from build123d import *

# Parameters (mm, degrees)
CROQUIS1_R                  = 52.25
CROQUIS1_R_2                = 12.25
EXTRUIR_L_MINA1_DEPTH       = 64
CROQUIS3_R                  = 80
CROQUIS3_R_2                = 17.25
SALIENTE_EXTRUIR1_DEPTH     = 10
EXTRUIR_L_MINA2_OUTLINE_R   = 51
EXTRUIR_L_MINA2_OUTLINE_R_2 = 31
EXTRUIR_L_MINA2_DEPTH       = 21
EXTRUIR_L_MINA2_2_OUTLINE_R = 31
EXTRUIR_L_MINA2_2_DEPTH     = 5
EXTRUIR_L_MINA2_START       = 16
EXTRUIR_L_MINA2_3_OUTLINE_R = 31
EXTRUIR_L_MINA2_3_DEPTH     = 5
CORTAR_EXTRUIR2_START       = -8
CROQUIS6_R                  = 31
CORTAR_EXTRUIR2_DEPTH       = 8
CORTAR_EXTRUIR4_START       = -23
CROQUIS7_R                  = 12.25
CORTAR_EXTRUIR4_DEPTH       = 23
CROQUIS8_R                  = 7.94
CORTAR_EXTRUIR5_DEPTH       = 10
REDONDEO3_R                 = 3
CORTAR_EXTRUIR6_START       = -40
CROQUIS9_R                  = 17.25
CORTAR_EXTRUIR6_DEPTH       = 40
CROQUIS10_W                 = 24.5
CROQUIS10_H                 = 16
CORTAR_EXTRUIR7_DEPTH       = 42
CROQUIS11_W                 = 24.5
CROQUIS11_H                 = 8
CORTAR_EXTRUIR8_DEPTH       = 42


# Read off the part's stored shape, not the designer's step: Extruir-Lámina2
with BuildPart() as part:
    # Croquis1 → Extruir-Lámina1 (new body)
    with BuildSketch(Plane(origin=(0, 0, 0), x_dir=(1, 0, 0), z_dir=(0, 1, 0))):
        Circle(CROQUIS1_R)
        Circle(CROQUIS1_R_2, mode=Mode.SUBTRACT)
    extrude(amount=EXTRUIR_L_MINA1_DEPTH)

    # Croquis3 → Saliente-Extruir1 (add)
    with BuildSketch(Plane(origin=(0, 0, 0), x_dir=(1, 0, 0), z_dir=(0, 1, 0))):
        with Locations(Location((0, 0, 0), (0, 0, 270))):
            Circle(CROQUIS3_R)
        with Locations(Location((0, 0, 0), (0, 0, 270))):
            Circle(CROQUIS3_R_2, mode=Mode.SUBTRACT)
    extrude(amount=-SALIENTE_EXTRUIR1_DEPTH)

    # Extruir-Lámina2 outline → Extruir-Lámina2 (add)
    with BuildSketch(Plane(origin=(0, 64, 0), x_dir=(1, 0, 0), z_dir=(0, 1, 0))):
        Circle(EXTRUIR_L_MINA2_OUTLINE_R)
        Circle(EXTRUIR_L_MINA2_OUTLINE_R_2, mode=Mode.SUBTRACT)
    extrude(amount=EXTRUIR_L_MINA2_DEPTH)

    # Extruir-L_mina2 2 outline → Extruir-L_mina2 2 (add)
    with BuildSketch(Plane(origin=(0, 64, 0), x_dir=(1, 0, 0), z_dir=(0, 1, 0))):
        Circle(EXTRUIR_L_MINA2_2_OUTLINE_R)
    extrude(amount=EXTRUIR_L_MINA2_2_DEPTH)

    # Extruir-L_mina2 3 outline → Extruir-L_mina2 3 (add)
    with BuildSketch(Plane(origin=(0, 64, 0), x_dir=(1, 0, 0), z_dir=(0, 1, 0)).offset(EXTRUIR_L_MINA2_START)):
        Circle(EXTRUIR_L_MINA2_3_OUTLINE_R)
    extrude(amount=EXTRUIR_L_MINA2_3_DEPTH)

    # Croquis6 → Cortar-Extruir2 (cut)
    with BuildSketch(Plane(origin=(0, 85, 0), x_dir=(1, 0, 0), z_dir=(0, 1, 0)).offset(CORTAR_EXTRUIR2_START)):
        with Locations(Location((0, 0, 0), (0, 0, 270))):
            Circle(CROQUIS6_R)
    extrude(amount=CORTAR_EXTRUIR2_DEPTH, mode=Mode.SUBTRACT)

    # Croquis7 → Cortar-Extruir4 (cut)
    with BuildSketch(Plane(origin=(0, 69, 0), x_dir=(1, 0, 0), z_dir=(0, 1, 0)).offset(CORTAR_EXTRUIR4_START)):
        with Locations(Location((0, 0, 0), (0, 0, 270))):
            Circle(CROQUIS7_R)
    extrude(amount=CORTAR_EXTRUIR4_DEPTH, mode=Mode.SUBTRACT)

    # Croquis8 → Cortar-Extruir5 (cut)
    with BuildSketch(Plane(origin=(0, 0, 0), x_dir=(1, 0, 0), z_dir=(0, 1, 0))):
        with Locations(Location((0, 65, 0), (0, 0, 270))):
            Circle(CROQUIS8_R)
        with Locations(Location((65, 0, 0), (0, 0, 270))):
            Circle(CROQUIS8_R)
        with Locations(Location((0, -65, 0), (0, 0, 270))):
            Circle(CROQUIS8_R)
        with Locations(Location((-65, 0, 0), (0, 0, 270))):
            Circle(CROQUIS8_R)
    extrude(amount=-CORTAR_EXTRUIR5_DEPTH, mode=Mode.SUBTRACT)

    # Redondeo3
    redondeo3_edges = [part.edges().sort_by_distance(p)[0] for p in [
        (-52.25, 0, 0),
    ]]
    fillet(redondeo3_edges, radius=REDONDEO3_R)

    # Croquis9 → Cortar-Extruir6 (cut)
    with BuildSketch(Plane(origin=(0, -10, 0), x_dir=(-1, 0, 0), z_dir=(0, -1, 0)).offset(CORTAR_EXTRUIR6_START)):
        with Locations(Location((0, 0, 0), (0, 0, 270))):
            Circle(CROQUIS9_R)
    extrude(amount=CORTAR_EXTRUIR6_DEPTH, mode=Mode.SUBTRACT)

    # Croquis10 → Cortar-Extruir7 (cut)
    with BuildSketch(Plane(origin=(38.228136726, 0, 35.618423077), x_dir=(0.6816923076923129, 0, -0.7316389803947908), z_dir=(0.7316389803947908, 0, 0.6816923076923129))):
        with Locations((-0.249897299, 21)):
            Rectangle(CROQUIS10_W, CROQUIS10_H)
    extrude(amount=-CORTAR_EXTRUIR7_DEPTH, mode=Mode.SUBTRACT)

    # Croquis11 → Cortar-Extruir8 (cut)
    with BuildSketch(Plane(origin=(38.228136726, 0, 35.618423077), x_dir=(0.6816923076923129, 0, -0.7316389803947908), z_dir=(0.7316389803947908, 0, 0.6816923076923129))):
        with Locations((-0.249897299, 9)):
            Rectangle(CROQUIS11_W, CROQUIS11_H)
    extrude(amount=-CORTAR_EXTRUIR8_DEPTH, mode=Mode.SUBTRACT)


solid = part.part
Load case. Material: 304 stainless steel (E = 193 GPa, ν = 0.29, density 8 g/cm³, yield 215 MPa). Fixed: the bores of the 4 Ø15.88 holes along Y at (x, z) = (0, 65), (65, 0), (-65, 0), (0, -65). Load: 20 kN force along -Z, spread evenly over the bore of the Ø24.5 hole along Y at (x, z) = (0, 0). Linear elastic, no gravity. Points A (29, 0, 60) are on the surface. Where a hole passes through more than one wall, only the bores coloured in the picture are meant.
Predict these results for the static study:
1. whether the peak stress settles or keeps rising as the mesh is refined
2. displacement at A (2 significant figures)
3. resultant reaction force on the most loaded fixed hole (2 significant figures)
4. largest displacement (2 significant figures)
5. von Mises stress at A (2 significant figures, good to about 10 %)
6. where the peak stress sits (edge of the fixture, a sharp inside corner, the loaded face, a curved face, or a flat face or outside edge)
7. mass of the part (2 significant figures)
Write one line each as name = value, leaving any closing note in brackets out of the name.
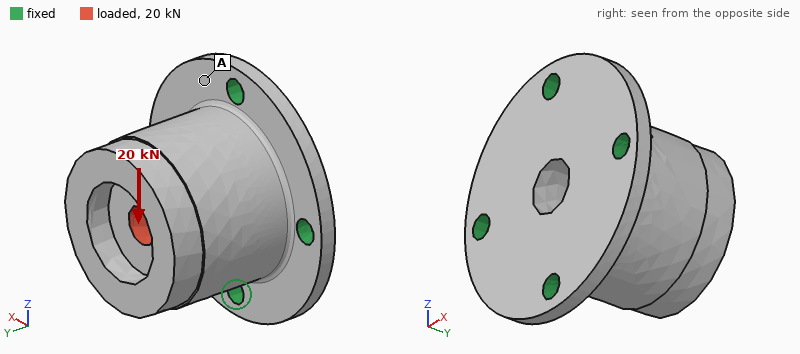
whether the peak stress settles or keeps rising as the mesh is refined = keeps rising
displacement at A = 4.2 µm
resultant reaction force on the most loaded fixed hole = 12 kN
largest displacement = 19 µm
von Mises stress at A = 7.1 MPa
where the peak stress sits = edge of the fixture
mass of the part = 6.3 kg
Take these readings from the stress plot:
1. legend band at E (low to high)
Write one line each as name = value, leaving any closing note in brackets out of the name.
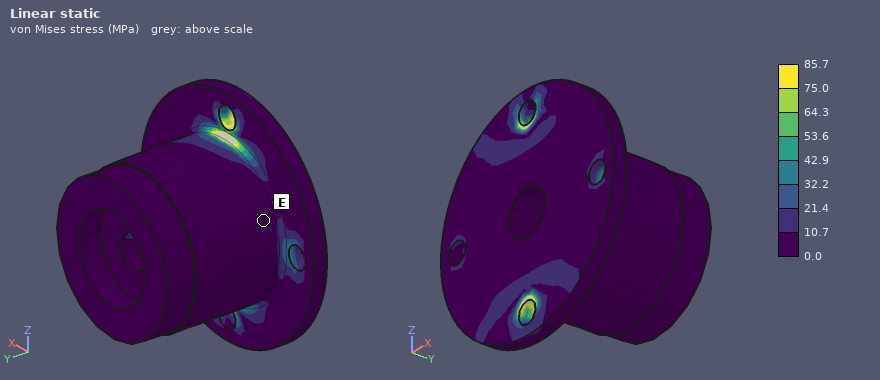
legend band at E = 0.0 to 10.7 MPa
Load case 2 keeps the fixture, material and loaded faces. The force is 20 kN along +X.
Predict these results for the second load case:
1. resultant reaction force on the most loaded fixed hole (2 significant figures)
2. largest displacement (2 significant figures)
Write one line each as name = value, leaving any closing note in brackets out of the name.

resultant reaction force on the most loaded fixed hole = 12 kN
largest displacement = 19 µm
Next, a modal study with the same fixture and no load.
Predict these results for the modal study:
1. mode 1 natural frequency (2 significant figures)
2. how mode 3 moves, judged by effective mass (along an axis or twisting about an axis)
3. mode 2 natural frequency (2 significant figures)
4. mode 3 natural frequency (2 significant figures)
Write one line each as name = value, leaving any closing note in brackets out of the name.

mode 1 natural frequency = 2900 Hz
how mode 3 moves, judged by effective mass = along Y
mode 2 natural frequency = 3000 Hz
mode 3 natural frequency = 4300 Hz
